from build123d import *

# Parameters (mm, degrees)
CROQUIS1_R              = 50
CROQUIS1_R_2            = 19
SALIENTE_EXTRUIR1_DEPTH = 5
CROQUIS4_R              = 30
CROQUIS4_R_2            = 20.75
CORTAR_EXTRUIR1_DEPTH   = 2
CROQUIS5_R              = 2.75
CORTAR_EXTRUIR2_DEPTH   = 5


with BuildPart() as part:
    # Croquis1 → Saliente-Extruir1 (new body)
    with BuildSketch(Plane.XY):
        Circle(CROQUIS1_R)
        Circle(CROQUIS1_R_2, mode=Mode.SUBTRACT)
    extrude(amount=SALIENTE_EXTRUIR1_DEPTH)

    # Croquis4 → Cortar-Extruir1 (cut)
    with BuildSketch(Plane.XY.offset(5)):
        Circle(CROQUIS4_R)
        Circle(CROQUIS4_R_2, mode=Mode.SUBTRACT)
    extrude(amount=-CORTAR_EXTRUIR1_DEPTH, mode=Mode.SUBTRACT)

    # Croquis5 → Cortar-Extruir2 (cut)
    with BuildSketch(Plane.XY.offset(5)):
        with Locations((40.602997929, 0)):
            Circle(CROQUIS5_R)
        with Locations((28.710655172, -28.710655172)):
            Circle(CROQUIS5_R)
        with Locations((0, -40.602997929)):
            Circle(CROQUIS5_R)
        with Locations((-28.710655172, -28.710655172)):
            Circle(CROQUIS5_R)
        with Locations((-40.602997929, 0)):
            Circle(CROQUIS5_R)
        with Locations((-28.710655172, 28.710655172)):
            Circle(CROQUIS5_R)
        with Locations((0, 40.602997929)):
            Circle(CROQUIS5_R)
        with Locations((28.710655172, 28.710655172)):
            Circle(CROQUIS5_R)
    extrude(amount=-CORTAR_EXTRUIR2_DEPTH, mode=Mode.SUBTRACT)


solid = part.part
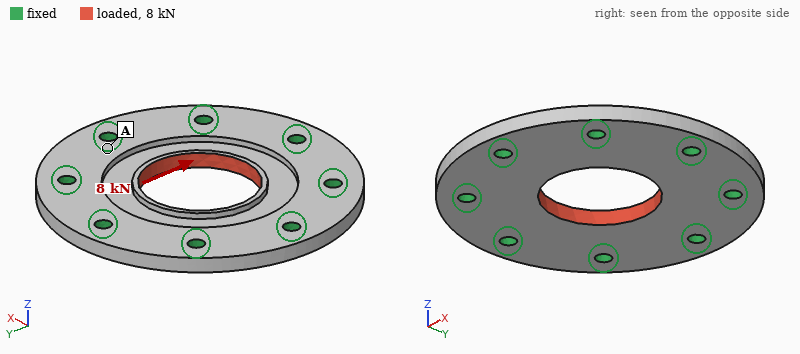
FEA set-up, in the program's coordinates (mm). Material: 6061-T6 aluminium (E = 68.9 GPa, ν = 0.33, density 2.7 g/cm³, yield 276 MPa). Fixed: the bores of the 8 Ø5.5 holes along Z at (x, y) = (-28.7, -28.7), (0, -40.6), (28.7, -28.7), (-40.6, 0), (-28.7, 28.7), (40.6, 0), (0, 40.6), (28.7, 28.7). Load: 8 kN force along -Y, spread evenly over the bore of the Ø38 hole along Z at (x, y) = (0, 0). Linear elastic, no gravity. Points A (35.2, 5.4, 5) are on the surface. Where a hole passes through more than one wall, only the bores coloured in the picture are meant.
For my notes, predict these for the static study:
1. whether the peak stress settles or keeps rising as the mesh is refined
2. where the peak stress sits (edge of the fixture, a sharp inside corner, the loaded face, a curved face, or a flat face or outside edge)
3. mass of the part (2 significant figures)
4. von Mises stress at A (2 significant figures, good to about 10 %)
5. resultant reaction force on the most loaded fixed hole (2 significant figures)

keeps rising
edge of the fixture
80 g
6.8 MPa
1.5 kN
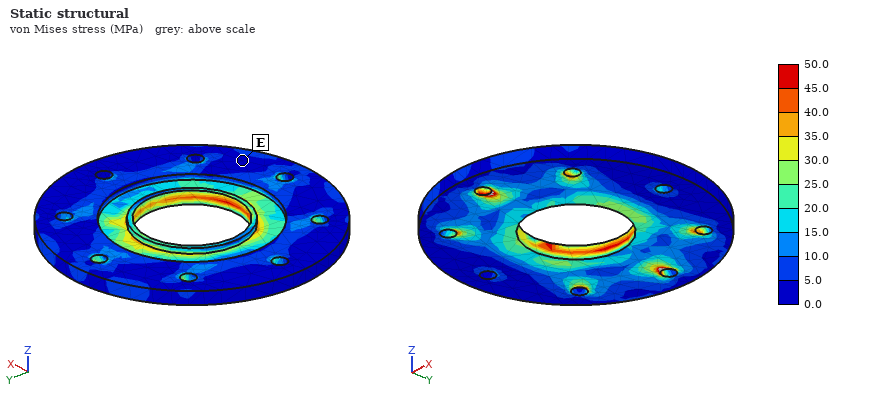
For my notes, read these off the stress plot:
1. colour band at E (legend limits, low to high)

0.0 to 5.0 MPa
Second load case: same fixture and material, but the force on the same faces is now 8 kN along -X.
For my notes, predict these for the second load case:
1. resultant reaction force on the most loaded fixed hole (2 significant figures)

1.5 kN
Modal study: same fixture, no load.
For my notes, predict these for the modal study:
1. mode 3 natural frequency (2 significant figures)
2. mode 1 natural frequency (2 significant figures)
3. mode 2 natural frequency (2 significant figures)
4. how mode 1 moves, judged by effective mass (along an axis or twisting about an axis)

13 kHz
11 kHz
13 kHz
along Z
